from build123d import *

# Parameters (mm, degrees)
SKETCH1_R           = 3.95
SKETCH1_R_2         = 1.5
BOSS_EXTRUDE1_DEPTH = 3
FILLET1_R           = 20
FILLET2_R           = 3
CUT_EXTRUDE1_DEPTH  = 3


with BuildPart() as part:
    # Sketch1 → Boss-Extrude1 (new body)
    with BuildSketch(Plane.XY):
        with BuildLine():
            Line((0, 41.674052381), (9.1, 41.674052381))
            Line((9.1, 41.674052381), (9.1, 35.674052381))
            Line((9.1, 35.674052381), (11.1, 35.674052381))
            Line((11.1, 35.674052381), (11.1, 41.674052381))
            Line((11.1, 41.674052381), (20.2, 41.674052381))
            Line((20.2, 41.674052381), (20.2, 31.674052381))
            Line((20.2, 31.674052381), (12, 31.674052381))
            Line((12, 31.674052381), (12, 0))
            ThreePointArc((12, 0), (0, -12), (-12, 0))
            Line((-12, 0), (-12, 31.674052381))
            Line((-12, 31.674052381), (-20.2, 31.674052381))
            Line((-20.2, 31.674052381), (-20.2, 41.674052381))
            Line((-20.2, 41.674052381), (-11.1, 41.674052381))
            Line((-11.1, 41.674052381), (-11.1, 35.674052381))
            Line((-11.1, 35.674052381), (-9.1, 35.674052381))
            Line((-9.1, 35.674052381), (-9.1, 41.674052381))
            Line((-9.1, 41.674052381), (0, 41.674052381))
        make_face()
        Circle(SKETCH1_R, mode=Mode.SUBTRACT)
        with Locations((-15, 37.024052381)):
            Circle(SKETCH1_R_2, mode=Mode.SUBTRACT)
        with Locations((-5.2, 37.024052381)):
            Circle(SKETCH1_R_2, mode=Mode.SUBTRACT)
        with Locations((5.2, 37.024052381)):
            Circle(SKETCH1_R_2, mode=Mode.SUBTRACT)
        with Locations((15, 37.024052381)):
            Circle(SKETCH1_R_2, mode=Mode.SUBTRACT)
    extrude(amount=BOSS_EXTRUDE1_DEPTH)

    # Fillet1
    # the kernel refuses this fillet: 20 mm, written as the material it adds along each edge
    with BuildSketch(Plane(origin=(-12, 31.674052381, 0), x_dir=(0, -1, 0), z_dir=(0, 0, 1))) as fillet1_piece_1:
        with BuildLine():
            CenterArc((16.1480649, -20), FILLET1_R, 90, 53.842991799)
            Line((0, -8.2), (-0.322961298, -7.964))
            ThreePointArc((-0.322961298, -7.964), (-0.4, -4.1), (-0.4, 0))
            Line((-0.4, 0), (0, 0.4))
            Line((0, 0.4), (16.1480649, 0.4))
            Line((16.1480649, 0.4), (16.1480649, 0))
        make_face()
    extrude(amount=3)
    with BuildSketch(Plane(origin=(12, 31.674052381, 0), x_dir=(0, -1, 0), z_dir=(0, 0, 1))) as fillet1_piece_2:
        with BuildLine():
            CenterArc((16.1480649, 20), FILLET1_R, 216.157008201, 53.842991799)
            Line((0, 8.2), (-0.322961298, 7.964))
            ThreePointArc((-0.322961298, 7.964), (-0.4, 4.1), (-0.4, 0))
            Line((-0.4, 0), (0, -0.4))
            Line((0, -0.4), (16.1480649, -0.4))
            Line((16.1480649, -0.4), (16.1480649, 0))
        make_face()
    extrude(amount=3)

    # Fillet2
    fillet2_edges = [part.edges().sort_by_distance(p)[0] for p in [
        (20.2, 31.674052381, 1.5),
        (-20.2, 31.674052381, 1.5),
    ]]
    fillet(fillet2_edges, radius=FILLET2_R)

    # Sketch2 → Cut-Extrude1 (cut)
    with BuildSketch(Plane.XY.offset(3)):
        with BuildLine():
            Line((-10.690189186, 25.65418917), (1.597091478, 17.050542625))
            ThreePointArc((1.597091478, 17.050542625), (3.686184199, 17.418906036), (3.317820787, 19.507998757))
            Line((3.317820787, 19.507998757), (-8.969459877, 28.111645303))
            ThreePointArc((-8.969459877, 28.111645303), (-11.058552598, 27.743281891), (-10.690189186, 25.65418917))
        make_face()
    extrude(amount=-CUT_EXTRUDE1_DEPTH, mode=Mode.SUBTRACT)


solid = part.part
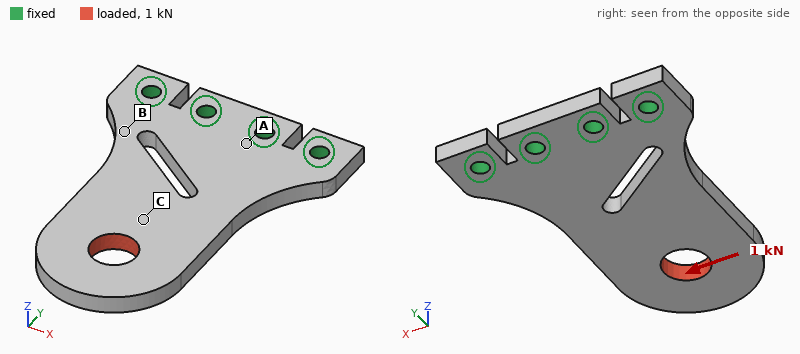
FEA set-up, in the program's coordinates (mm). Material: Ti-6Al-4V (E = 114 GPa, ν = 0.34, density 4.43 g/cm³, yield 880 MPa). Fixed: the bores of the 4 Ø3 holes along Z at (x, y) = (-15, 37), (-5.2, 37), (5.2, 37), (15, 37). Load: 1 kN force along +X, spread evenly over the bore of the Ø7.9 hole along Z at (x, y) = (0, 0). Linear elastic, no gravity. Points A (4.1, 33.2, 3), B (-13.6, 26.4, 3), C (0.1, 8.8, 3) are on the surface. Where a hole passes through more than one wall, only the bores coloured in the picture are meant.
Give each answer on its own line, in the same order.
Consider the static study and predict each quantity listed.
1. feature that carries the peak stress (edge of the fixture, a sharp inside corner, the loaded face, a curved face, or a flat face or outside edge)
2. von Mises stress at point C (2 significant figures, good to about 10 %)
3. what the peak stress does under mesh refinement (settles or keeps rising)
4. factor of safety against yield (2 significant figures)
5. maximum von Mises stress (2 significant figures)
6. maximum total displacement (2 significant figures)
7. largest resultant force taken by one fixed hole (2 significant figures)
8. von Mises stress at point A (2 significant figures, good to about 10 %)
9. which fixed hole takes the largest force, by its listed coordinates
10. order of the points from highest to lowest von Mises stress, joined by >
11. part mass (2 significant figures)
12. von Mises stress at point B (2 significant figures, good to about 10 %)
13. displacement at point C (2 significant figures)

a curved face
46 MPa
settles
4.1
220 MPa
55 µm
1.2 kN
15 MPa
(-15, 37)
B > C > A
17 g
85 MPa
24 µm
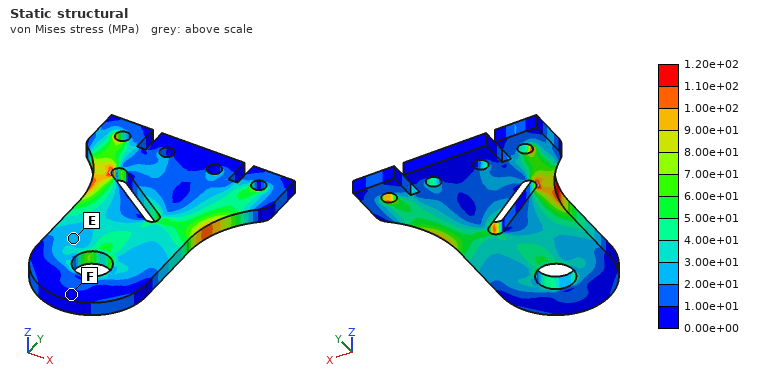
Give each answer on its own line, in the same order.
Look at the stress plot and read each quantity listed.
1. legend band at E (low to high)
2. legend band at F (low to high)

2.00e+01 to 3.00e+01 MPa
0.00e+00 to 1.00e+01 MPa
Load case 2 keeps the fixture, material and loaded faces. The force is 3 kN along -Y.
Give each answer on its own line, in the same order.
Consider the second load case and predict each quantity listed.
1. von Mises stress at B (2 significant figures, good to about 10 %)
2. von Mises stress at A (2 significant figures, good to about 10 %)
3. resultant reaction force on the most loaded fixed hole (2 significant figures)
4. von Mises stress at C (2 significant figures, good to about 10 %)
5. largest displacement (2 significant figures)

72 MPa
33 MPa
1.0 kN
35 MPa
27 µm
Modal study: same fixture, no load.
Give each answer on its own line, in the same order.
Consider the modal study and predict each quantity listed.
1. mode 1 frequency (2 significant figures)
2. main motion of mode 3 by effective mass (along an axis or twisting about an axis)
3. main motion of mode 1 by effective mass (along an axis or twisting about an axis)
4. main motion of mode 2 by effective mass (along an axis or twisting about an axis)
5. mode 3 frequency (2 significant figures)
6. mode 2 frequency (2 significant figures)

1200 Hz
along Z
along Z
twisting about Y
6900 Hz
5000 Hz
